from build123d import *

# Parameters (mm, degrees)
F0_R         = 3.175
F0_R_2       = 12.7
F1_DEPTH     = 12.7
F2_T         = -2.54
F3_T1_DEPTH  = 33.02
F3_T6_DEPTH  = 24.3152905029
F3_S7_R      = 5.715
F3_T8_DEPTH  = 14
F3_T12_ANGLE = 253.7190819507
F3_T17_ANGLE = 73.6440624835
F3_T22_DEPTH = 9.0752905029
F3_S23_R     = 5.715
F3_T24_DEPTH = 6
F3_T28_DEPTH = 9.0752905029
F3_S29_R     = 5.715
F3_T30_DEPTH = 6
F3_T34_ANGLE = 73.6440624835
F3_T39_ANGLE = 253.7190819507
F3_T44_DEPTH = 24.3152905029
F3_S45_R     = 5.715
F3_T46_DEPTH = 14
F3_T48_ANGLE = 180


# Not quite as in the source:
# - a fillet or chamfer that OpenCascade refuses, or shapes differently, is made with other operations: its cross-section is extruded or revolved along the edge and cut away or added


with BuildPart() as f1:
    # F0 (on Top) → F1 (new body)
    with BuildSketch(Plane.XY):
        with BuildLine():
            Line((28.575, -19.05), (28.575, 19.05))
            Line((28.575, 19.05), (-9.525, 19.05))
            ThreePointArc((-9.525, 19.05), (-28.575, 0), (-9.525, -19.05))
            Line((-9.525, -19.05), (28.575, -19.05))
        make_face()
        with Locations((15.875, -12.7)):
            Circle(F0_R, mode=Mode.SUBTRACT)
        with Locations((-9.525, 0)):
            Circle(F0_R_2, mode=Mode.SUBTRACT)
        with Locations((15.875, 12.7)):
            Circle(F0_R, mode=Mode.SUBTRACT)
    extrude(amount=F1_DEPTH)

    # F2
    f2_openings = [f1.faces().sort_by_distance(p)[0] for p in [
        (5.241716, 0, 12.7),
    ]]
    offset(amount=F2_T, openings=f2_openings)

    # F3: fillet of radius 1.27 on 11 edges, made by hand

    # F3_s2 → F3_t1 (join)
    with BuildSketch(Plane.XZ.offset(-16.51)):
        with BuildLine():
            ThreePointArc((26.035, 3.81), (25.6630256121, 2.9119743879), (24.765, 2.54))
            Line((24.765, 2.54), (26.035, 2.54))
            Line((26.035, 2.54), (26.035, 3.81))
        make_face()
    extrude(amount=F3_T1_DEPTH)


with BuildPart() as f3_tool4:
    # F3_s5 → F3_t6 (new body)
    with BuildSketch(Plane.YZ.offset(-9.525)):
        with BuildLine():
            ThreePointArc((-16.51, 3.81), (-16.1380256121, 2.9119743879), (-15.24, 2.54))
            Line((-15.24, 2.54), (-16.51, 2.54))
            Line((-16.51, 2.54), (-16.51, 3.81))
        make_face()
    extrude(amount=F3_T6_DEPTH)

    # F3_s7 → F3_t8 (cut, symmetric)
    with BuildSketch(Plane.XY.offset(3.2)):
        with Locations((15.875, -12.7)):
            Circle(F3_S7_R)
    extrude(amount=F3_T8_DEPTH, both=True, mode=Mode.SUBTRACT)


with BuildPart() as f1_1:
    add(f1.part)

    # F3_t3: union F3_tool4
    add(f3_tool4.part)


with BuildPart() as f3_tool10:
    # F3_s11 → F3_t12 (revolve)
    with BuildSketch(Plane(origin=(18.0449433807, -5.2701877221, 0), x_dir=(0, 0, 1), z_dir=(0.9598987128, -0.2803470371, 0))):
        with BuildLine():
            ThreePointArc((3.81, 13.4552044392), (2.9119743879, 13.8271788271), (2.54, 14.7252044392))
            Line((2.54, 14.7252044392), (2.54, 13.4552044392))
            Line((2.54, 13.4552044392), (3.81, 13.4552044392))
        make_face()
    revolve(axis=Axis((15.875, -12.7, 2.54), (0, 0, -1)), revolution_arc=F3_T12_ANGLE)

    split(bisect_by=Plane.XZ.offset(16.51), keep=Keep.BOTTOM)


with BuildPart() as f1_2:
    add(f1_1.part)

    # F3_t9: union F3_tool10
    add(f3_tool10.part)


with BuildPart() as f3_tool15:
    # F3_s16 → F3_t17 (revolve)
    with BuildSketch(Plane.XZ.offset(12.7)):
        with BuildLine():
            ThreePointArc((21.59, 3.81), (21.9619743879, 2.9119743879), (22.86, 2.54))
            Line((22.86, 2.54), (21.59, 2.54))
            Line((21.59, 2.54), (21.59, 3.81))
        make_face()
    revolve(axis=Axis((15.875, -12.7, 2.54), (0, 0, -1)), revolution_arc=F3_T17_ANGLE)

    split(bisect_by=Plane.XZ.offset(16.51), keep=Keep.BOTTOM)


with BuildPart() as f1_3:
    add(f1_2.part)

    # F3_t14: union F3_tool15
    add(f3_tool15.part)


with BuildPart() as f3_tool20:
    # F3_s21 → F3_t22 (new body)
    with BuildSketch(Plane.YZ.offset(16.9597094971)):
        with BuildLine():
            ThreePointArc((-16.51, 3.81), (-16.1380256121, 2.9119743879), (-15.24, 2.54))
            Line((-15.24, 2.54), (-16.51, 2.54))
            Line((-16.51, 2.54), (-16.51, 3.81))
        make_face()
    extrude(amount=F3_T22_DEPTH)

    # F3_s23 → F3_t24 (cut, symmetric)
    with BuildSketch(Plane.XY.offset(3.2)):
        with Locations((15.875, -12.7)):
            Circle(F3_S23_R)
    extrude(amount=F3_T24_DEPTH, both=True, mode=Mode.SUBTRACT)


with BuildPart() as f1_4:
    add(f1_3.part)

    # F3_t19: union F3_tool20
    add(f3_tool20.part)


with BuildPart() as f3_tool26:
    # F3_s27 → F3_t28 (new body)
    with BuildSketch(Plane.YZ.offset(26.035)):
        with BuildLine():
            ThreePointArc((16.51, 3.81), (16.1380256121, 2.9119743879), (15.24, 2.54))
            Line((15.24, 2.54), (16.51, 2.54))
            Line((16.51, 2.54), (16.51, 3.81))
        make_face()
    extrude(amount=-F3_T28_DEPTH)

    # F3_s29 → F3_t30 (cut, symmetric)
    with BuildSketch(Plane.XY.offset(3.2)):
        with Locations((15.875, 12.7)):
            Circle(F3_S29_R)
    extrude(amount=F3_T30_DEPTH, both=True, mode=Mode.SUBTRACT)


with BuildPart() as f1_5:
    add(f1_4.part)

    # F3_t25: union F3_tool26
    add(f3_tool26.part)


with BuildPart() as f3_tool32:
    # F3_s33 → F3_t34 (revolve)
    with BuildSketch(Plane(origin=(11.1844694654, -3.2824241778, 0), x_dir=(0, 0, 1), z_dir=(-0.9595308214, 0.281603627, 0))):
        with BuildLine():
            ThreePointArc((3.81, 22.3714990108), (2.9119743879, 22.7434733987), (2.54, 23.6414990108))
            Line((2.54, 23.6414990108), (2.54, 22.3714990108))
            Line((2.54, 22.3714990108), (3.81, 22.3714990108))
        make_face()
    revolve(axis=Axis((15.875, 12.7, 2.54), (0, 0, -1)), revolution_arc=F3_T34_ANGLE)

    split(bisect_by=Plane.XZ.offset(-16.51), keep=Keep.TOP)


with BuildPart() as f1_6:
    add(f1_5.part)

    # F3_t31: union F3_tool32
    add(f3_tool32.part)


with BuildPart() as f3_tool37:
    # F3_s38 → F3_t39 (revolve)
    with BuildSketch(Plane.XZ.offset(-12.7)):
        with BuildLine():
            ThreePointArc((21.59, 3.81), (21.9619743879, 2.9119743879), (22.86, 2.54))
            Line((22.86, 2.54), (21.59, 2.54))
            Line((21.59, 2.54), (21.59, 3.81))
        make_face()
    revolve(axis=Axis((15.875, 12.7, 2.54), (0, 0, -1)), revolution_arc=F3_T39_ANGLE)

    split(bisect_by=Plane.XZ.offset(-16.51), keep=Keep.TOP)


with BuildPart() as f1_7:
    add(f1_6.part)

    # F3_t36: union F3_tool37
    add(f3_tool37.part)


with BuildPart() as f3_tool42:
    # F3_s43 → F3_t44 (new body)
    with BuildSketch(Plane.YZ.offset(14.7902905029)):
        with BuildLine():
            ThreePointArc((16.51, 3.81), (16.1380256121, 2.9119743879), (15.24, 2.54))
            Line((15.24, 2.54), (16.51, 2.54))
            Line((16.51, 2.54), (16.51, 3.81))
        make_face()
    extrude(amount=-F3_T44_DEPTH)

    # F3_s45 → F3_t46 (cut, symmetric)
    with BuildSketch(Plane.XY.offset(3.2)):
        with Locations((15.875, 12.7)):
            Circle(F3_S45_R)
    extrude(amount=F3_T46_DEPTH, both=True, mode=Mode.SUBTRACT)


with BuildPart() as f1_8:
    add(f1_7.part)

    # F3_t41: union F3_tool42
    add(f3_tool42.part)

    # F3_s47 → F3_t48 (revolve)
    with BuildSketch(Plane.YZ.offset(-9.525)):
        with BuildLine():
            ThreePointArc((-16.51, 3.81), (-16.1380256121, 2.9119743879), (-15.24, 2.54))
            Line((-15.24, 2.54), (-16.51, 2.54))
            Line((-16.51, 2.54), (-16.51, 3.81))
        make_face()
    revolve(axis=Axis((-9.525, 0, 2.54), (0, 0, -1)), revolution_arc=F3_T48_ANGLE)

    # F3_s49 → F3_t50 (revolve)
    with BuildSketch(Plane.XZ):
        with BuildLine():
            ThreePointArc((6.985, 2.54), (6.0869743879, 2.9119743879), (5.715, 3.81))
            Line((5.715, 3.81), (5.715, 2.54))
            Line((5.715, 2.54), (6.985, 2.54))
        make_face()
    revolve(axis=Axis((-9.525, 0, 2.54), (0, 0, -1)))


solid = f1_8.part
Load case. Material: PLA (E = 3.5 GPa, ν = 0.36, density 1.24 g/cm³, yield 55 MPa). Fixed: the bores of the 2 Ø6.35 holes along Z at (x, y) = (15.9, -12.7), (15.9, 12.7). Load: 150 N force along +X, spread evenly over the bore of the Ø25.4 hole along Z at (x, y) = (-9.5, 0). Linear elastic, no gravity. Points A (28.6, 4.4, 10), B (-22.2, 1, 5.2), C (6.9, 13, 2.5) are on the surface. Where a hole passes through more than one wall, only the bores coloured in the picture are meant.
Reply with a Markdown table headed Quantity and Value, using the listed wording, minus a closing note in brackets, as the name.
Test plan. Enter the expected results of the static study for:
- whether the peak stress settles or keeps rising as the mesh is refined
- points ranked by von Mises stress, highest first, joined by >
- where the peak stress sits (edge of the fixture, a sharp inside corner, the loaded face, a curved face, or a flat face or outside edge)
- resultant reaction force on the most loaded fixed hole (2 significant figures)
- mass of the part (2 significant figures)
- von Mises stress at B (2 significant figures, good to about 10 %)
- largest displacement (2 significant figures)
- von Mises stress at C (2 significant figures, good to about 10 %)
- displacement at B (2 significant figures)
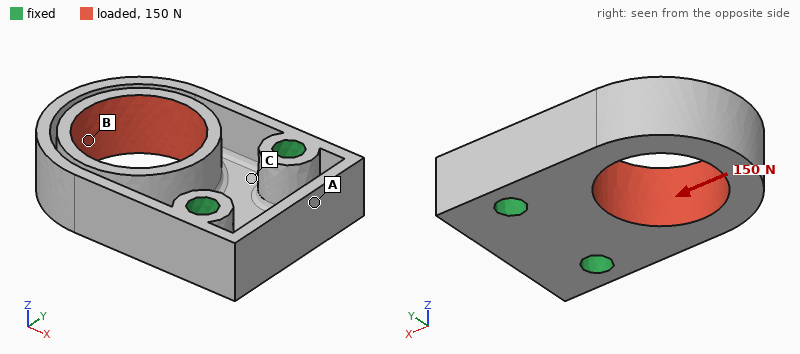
| Quantity | Value |
|---|---|
| whether the peak stress settles or keeps rising as the mesh is refined | keeps rising |
| points ranked by von Mises stress, highest first, joined by > | C > B > A |
| where the peak stress sits | a sharp inside corner |
| resultant reaction force on the most loaded fixed hole | 75 N |
| mass of the part | 14 g |
| von Mises stress at B | 0.94 MPa |
| largest displacement | 98 µm |
| von Mises stress at C | 1.6 MPa |
| displacement at B | 69 µm |
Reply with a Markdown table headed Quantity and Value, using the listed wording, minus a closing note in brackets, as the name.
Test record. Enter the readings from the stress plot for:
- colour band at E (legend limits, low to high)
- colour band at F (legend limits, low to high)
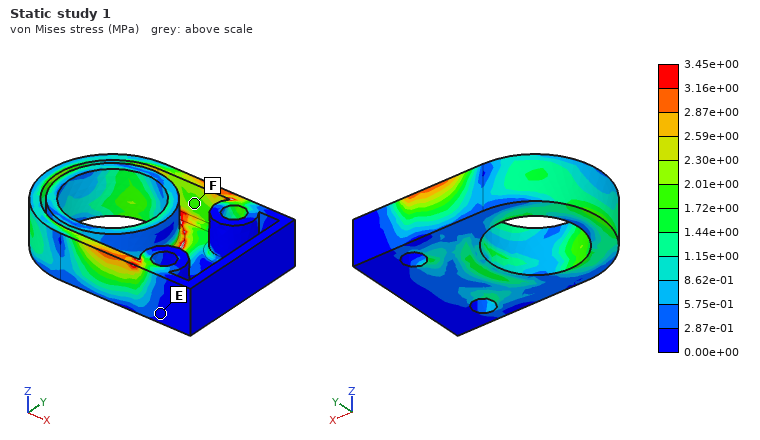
| Quantity | Value |
|---|---|
| colour band at E | 0.00e+00 to 2.87e-01 MPa |
| colour band at F | 1.72e+00 to 2.01e+00 MPa |
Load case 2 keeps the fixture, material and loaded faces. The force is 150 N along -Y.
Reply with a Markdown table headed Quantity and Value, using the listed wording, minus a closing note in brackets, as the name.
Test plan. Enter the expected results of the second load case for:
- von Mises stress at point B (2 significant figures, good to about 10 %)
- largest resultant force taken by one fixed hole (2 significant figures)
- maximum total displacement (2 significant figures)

| Quantity | Value |
|---|---|
| von Mises stress at point B | 2.4 MPa |
| largest resultant force taken by one fixed hole | 140 N |
| maximum total displacement | 0.22 mm |
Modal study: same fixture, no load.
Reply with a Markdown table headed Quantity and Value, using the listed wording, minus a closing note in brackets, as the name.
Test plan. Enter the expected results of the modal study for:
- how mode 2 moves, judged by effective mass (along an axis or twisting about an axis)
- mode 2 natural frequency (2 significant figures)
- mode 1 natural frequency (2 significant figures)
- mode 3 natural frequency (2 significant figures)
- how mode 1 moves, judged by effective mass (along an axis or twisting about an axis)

| Quantity | Value |
|---|---|
| how mode 2 moves, judged by effective mass | along Y |
| mode 2 natural frequency | 1700 Hz |
| mode 1 natural frequency | 1200 Hz |
| mode 3 natural frequency | 3000 Hz |
| how mode 1 moves, judged by effective mass | along Z |
